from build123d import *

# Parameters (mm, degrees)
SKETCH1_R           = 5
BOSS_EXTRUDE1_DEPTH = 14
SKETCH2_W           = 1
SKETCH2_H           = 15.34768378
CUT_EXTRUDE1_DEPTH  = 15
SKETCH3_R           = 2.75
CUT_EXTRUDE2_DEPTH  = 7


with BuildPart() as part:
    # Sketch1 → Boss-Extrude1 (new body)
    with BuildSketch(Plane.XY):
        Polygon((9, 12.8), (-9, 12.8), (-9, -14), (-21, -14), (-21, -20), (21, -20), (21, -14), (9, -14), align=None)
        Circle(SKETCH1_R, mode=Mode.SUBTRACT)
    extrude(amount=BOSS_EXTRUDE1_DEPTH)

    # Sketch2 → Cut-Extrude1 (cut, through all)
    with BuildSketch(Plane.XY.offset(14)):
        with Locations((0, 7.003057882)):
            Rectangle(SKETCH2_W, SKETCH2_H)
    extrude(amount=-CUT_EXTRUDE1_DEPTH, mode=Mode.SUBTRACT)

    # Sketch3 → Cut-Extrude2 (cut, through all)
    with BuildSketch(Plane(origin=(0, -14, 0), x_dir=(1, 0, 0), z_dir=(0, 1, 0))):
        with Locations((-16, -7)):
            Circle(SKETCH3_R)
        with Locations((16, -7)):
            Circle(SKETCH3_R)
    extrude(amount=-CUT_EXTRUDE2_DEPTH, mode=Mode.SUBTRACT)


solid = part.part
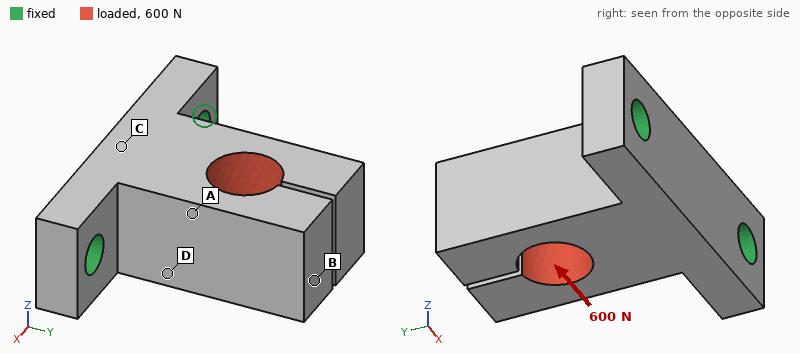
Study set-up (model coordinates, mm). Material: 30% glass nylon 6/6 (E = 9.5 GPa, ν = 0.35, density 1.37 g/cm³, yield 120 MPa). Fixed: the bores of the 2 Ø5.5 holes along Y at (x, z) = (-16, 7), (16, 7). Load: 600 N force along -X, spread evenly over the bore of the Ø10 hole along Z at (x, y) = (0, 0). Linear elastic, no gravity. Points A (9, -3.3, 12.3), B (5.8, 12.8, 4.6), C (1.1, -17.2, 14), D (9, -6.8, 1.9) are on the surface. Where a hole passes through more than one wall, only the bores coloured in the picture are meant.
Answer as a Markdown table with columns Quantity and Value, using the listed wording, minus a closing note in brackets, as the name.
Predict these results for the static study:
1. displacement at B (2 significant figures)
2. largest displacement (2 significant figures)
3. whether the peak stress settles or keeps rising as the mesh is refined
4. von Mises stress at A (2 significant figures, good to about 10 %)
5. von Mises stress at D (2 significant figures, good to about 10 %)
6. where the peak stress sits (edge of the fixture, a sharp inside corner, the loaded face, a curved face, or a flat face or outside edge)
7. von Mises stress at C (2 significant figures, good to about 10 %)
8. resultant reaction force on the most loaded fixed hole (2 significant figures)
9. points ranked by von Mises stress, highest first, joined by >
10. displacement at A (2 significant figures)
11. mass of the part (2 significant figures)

| Quantity | Value |
|---|---|
| displacement at B | 0.18 mm |
| largest displacement | 0.18 mm |
| whether the peak stress settles or keeps rising as the mesh is refined | keeps rising |
| von Mises stress at A | 16 MPa |
| von Mises stress at D | 12 MPa |
| where the peak stress sits | edge of the fixture |
| von Mises stress at C | 4.7 MPa |
| resultant reaction force on the most loaded fixed hole | 520 N |
| points ranked by von Mises stress, highest first, joined by > | A > D > C > B |
| displacement at A | 0.053 mm |
| mass of the part | 12 g |
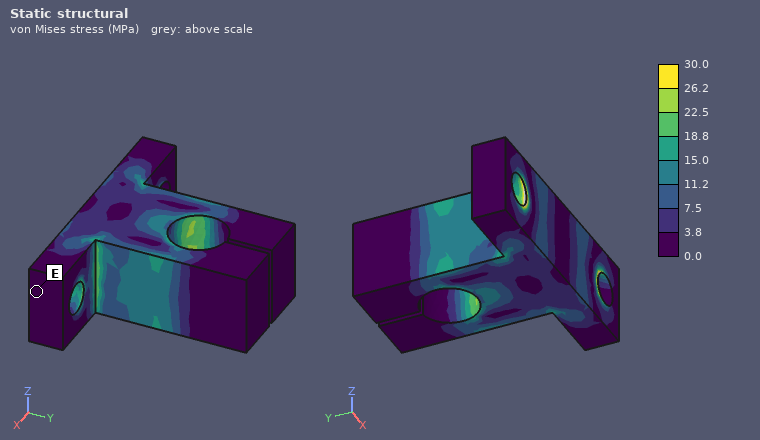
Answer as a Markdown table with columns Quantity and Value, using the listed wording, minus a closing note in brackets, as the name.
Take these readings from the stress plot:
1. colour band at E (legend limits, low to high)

| Quantity | Value |
|---|---|
| colour band at E | 0.0 to 3.8 MPa |
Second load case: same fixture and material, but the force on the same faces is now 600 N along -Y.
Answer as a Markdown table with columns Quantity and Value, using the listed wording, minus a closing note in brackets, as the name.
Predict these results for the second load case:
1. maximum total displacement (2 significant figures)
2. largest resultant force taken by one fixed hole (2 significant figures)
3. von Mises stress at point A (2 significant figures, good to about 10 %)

| Quantity | Value |
|---|---|
| maximum total displacement | 91 µm |
| largest resultant force taken by one fixed hole | 320 N |
| von Mises stress at point A | 6.9 MPa |
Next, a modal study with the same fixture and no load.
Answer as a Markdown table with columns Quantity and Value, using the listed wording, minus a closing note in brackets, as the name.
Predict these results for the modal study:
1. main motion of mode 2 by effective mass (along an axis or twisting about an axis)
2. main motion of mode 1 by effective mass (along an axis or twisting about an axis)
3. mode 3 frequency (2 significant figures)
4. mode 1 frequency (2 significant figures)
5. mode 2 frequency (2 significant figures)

| Quantity | Value |
|---|---|
| main motion of mode 2 by effective mass | along X |
| main motion of mode 1 by effective mass | along Z |
| mode 3 frequency | 3800 Hz |
| mode 1 frequency | 2600 Hz |
| mode 2 frequency | 3400 Hz |
